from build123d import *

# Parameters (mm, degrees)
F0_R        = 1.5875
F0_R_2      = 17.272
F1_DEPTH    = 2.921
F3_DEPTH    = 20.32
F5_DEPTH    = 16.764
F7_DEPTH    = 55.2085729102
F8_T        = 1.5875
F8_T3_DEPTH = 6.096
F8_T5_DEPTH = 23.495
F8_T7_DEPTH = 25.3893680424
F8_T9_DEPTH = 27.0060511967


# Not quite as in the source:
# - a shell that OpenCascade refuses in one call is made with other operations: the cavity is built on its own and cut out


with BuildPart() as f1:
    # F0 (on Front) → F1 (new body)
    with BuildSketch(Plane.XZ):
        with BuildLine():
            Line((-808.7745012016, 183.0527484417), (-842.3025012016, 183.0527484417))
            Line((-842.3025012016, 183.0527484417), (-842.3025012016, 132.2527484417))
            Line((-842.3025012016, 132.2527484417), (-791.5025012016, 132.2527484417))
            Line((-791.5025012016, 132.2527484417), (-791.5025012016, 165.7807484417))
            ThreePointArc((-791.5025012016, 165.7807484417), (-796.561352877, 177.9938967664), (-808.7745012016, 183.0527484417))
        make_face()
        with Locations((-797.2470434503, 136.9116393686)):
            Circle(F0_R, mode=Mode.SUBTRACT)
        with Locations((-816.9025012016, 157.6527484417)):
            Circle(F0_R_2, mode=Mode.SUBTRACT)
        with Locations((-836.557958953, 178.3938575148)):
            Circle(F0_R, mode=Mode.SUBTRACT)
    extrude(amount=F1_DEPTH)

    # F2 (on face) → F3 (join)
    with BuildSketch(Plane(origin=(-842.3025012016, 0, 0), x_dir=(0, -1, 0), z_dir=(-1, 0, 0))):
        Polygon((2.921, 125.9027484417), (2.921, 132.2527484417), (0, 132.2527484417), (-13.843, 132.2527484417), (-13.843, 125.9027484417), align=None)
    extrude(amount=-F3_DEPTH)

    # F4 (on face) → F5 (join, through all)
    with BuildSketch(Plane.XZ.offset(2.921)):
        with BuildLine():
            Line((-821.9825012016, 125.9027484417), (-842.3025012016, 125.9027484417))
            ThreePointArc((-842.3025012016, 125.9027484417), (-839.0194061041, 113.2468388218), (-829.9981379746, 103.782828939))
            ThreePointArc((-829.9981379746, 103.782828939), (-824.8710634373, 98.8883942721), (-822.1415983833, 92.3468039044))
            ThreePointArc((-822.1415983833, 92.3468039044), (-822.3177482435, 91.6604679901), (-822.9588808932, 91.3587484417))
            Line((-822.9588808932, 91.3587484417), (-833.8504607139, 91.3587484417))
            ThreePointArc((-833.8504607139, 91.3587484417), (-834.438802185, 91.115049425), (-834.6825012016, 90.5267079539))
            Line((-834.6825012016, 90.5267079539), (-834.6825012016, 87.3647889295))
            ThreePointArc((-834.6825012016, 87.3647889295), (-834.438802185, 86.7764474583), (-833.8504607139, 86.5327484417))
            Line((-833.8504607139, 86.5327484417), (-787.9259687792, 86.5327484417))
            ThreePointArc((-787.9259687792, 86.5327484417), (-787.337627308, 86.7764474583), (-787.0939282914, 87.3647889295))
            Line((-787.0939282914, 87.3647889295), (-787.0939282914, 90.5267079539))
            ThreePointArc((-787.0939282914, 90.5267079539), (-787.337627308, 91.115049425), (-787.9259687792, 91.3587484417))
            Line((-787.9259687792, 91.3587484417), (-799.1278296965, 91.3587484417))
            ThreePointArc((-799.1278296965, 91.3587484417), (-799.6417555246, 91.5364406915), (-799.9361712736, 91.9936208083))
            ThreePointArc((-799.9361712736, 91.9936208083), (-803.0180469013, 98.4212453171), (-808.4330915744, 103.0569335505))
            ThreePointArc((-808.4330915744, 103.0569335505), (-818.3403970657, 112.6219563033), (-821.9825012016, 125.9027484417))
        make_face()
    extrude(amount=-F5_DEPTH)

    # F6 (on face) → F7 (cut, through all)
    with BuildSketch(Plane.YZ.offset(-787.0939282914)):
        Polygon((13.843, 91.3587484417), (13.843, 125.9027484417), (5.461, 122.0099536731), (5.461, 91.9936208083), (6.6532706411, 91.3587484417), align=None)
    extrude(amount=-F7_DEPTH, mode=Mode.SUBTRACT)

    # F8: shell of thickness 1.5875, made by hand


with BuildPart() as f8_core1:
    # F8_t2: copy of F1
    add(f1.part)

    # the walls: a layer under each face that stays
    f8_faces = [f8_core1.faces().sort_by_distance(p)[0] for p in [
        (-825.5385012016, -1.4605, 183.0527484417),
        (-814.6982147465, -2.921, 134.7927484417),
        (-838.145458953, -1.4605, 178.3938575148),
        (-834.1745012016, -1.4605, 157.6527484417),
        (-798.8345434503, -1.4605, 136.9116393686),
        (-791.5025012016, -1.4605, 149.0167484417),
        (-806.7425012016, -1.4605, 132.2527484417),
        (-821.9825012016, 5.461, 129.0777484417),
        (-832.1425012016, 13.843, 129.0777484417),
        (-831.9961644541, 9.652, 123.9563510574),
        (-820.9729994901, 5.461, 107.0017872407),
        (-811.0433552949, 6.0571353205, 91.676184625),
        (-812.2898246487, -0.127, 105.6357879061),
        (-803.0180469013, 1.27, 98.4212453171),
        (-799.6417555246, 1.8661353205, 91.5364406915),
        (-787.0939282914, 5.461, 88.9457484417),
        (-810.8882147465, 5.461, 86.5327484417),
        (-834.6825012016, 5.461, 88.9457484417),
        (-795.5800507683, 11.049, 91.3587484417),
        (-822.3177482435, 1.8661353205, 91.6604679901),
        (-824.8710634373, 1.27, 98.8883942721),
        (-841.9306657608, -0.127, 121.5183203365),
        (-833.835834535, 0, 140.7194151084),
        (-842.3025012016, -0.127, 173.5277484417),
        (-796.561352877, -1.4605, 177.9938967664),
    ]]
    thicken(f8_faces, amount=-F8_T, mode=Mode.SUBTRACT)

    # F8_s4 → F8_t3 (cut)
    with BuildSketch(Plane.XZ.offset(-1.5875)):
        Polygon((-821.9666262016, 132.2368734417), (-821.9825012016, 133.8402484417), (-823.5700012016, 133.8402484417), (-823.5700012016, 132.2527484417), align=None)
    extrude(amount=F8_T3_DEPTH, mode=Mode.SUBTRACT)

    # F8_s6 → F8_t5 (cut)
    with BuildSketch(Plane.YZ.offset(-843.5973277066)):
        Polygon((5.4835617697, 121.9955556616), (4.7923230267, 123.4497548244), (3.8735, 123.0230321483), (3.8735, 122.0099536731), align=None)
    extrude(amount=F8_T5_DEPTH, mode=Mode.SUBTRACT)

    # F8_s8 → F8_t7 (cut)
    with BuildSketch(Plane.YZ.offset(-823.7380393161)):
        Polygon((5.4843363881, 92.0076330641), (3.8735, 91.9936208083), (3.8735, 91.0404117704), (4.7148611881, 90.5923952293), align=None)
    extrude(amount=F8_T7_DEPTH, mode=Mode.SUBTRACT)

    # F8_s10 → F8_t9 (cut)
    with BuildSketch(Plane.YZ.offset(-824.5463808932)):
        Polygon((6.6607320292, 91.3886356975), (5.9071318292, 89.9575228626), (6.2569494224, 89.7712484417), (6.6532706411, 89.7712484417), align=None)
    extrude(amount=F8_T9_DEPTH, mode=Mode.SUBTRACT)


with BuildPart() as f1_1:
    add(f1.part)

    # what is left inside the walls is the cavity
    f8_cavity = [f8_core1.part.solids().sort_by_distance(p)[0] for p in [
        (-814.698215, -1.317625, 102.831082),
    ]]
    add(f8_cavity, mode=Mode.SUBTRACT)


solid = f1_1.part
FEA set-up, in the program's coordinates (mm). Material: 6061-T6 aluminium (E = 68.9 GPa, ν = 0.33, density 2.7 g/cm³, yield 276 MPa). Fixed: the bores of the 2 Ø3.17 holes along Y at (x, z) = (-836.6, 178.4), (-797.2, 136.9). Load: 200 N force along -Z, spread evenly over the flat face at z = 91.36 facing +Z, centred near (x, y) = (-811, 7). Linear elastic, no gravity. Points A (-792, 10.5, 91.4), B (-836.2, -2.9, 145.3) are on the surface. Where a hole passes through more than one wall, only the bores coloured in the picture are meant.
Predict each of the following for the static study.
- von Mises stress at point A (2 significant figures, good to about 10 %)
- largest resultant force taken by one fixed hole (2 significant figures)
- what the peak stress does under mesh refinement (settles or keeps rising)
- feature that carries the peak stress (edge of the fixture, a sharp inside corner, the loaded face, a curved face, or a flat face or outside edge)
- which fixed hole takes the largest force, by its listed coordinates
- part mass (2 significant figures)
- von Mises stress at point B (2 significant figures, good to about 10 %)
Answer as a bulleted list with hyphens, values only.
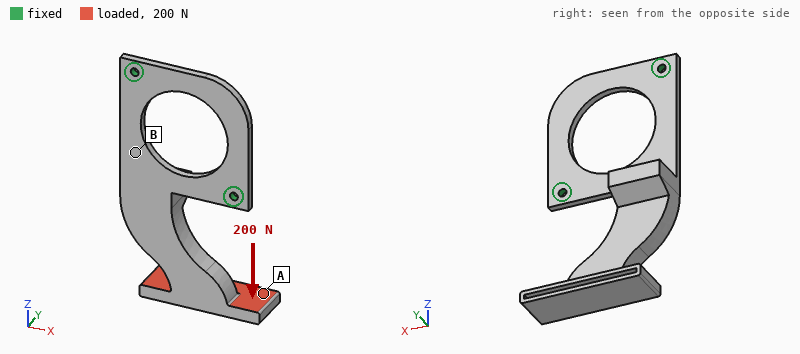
- 12 MPa
- 140 N
- keeps rising
- a sharp inside corner
- (-797.2, 136.9)
- 30 g
- 42 MPa
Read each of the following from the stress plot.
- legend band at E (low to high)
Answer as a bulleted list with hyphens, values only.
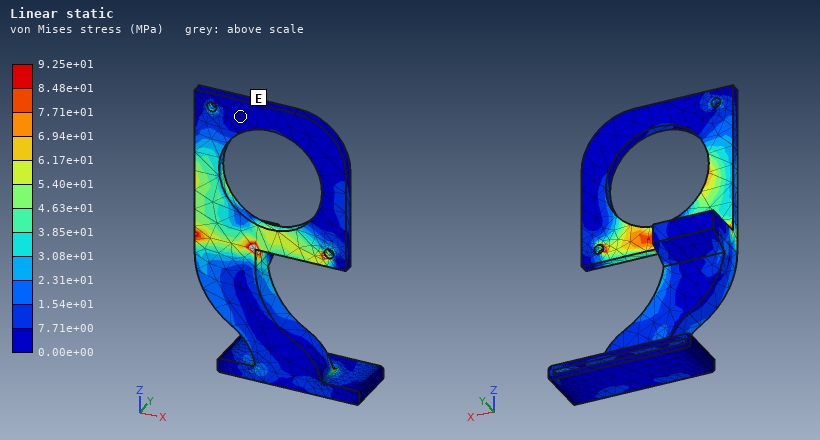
- 0.00e+00 to 7.71e+00 MPa
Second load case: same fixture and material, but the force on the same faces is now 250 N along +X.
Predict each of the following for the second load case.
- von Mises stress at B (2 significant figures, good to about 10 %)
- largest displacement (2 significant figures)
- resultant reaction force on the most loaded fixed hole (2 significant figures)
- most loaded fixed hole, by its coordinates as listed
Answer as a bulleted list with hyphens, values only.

- 44 MPa
- 0.76 mm
- 440 N
- (-797.2, 136.9)
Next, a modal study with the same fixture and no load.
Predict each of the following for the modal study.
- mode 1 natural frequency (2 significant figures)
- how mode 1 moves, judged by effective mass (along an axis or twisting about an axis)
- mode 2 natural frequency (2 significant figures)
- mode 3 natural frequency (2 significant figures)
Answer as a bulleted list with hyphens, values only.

- 290 Hz
- along Y
- 810 Hz
- 1600 Hz
